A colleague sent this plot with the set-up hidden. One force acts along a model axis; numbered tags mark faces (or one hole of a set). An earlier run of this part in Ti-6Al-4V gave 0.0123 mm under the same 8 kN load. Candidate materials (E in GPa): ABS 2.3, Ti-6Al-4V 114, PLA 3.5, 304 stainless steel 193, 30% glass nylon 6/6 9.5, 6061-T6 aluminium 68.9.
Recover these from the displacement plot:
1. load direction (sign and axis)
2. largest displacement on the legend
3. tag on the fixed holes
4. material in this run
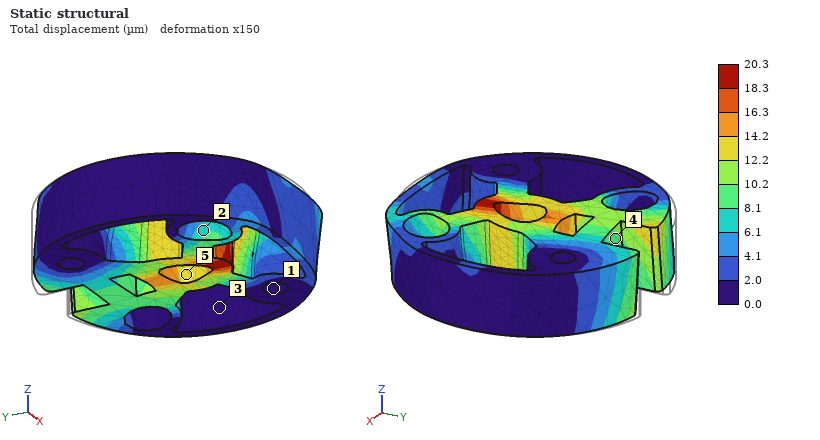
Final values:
-Y
20.3 µm
1
6061-T6 aluminium
